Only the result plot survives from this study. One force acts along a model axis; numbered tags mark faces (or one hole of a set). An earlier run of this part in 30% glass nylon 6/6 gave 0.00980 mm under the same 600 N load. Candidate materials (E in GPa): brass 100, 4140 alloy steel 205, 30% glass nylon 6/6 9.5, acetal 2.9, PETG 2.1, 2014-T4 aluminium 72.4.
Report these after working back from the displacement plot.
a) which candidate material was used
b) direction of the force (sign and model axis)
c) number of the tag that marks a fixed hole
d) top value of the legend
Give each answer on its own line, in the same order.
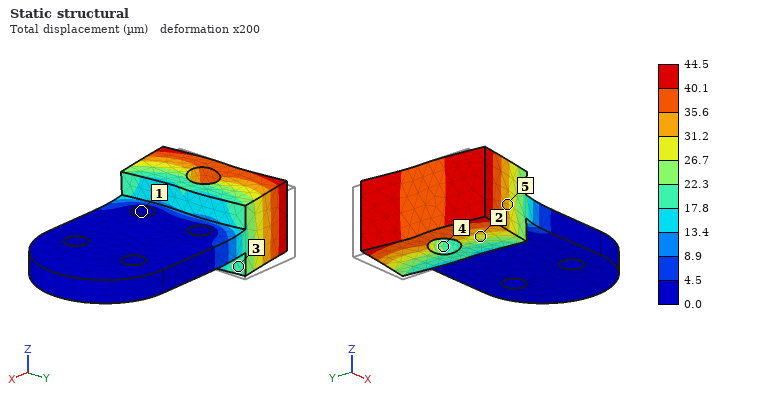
PETG
-Y
1
44.5 µm
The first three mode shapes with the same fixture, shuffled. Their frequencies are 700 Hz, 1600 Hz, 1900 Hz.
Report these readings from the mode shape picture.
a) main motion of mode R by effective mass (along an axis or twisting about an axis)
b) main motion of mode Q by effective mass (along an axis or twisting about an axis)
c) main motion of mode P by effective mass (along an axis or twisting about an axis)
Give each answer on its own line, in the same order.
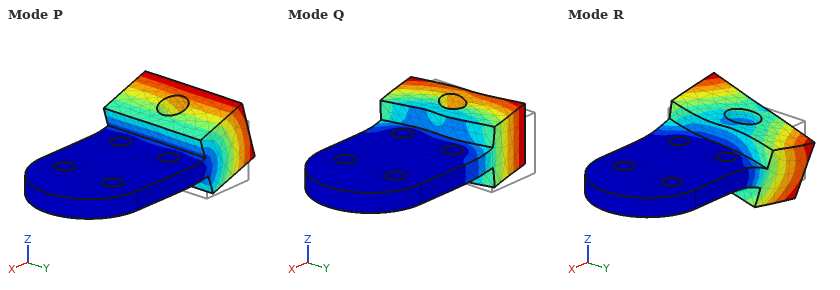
twisting about X
along Y
along Z
